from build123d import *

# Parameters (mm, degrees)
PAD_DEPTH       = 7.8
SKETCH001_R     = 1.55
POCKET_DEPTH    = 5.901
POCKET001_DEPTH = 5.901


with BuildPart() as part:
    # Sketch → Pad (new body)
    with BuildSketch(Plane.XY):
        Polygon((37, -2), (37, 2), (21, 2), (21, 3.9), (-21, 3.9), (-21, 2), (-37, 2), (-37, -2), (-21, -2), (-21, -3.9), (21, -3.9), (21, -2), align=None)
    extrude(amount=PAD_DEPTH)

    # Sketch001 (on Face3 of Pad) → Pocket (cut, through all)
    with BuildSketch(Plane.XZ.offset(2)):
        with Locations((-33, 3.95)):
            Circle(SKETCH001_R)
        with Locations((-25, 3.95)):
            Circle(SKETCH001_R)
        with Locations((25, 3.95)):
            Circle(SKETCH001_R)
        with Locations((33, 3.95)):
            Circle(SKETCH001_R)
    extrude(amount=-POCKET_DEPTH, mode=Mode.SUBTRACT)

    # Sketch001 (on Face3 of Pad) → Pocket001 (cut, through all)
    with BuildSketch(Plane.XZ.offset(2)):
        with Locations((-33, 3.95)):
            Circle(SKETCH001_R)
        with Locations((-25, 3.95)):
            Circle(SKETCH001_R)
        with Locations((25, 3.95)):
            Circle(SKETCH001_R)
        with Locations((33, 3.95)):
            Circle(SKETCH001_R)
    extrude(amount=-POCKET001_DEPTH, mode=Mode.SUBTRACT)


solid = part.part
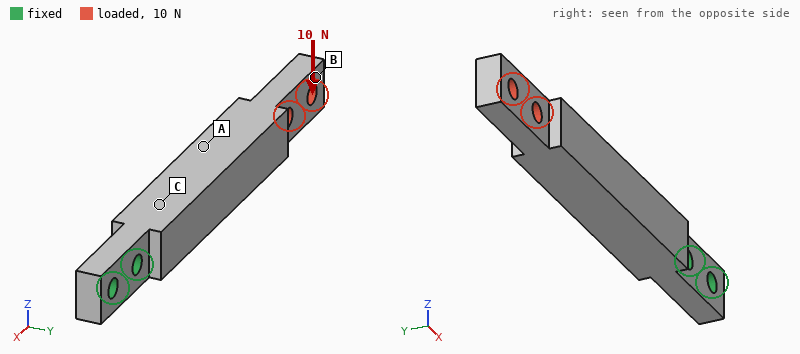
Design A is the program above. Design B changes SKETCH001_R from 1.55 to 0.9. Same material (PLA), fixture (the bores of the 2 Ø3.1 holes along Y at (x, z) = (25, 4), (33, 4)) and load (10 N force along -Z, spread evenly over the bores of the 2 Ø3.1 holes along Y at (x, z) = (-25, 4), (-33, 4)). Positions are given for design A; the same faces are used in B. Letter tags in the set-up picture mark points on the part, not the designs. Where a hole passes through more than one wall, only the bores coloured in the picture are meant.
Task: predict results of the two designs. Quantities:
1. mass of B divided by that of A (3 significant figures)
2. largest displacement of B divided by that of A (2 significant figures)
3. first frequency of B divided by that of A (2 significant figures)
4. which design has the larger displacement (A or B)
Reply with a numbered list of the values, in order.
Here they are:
1. 1.02
2. 1.1
3. 0.90
4. B
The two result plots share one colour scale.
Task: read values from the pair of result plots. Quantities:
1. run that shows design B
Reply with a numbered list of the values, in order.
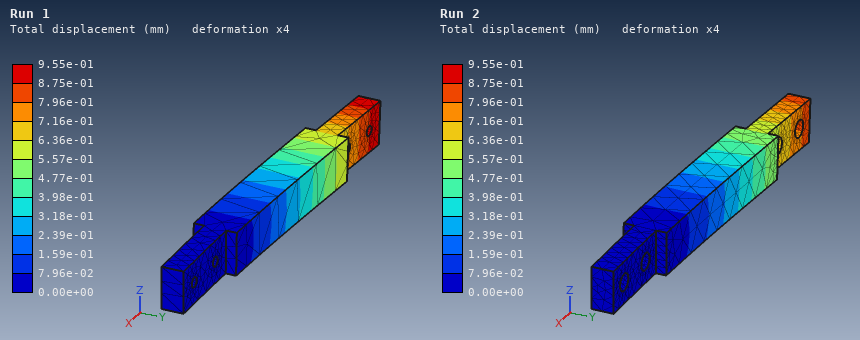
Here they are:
1. Run 1
